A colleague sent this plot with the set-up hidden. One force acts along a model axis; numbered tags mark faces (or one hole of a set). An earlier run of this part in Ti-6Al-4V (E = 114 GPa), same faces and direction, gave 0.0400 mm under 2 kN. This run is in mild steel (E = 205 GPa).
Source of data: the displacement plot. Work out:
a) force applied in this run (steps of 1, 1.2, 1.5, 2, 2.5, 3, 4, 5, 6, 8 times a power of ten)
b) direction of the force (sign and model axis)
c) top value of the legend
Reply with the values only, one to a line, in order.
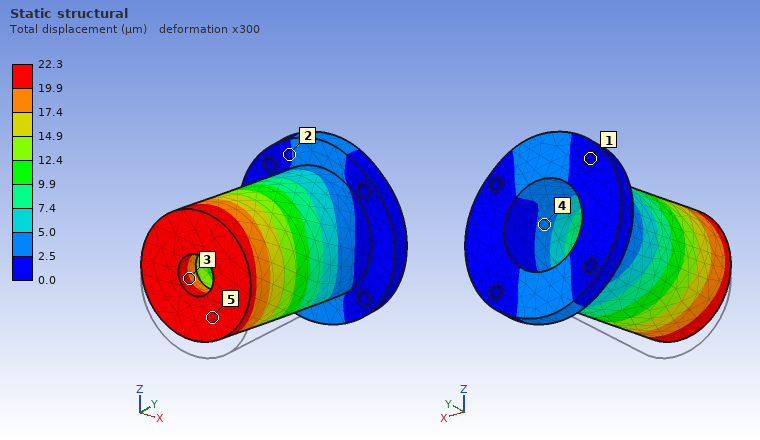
2 kN
+Z
22.3 µm
